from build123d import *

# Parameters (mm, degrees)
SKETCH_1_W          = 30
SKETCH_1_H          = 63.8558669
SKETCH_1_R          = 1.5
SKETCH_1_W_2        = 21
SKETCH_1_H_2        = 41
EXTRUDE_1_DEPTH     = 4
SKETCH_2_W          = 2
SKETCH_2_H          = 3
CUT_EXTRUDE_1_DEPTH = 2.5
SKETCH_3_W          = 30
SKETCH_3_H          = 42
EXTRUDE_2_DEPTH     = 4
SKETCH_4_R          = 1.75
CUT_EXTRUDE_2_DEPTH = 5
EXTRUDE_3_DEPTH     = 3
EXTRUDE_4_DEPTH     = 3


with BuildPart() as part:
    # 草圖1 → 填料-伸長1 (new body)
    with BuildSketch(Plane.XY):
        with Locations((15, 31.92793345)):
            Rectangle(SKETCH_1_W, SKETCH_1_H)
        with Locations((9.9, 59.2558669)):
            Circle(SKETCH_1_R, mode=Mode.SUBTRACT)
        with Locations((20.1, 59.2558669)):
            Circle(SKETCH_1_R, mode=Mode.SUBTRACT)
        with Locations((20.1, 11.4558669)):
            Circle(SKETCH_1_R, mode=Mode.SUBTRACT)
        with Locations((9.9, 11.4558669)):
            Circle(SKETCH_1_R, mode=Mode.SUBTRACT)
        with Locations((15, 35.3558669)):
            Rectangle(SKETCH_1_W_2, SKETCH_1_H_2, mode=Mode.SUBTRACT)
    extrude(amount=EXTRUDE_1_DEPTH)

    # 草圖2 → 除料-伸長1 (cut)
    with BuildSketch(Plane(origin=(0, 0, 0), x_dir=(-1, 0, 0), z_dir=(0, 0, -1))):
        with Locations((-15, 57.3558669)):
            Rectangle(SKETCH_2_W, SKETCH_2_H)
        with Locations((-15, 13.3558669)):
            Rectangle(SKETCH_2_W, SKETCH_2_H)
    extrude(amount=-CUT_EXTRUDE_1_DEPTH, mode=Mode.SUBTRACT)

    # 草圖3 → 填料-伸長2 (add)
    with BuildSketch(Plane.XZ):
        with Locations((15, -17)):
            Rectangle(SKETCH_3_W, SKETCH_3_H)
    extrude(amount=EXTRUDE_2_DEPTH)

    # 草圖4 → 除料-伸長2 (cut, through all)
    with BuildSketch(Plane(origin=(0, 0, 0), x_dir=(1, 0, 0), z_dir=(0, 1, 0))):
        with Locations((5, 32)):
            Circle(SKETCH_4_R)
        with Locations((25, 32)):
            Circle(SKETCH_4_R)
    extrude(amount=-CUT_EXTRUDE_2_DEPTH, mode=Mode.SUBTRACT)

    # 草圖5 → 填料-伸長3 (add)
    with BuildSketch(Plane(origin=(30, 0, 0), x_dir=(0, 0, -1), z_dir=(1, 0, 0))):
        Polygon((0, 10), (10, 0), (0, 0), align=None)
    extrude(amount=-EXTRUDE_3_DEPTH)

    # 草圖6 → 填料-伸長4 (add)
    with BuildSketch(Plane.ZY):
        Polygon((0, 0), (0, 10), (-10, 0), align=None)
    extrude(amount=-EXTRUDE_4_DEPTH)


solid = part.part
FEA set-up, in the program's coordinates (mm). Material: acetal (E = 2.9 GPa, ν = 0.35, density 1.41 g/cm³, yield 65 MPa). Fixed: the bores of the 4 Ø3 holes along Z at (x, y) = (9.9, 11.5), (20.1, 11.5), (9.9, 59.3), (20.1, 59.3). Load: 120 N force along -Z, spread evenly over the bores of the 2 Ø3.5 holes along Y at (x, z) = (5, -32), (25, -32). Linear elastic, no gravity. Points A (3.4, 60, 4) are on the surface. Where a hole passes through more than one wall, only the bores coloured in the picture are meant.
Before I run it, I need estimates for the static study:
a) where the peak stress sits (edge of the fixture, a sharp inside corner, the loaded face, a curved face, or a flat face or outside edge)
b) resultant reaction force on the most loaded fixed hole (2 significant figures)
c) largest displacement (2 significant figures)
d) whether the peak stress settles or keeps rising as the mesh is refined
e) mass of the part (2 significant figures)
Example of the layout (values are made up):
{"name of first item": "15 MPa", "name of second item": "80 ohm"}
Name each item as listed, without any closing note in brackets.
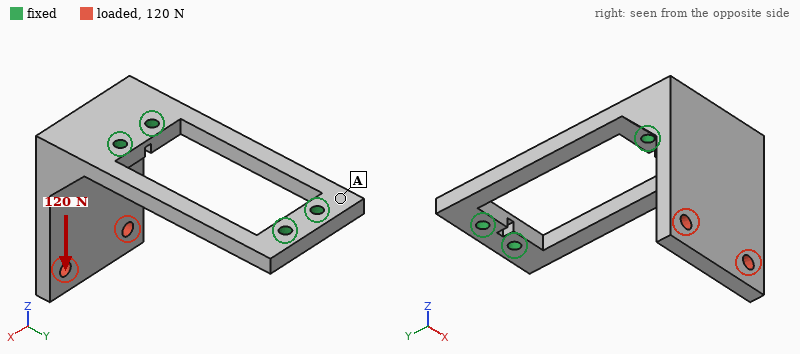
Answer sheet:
{"where the peak stress sits": "edge of the fixture", "resultant reaction force on the most loaded fixed hole": "62 N", "largest displacement": "0.83 mm", "whether the peak stress settles or keeps rising as the mesh is refined": "keeps rising", "mass of the part": "13 g"}
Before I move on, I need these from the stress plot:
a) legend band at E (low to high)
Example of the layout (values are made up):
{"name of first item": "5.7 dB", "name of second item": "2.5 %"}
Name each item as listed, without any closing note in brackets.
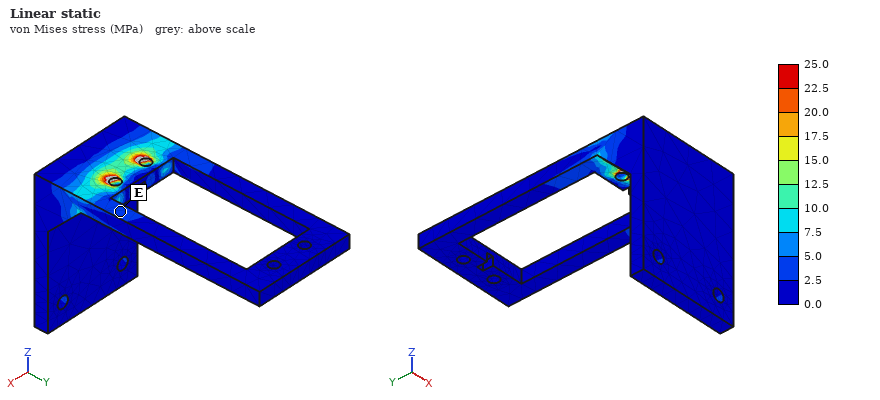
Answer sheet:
{"legend band at E": "2.5 to 5.0 MPa"}
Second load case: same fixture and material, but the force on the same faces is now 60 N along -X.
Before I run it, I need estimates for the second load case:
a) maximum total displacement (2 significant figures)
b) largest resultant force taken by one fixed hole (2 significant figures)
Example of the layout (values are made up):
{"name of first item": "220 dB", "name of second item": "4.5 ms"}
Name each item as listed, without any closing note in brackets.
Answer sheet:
{"maximum total displacement": "0.83 mm", "largest resultant force taken by one fixed hole": "130 N"}
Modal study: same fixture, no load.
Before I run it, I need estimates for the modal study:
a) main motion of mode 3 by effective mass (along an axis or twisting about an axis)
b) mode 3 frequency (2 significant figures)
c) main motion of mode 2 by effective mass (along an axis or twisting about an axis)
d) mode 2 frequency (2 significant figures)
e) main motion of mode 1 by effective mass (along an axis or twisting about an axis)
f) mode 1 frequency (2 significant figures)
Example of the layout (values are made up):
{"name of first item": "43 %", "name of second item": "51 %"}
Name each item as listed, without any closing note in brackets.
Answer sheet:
{"main motion of mode 3 by effective mass": "along Z", "mode 3 frequency": "1800 Hz", "main motion of mode 2 by effective mass": "along X", "mode 2 frequency": "810 Hz", "main motion of mode 1 by effective mass": "along Y", "mode 1 frequency": "490 Hz"}
